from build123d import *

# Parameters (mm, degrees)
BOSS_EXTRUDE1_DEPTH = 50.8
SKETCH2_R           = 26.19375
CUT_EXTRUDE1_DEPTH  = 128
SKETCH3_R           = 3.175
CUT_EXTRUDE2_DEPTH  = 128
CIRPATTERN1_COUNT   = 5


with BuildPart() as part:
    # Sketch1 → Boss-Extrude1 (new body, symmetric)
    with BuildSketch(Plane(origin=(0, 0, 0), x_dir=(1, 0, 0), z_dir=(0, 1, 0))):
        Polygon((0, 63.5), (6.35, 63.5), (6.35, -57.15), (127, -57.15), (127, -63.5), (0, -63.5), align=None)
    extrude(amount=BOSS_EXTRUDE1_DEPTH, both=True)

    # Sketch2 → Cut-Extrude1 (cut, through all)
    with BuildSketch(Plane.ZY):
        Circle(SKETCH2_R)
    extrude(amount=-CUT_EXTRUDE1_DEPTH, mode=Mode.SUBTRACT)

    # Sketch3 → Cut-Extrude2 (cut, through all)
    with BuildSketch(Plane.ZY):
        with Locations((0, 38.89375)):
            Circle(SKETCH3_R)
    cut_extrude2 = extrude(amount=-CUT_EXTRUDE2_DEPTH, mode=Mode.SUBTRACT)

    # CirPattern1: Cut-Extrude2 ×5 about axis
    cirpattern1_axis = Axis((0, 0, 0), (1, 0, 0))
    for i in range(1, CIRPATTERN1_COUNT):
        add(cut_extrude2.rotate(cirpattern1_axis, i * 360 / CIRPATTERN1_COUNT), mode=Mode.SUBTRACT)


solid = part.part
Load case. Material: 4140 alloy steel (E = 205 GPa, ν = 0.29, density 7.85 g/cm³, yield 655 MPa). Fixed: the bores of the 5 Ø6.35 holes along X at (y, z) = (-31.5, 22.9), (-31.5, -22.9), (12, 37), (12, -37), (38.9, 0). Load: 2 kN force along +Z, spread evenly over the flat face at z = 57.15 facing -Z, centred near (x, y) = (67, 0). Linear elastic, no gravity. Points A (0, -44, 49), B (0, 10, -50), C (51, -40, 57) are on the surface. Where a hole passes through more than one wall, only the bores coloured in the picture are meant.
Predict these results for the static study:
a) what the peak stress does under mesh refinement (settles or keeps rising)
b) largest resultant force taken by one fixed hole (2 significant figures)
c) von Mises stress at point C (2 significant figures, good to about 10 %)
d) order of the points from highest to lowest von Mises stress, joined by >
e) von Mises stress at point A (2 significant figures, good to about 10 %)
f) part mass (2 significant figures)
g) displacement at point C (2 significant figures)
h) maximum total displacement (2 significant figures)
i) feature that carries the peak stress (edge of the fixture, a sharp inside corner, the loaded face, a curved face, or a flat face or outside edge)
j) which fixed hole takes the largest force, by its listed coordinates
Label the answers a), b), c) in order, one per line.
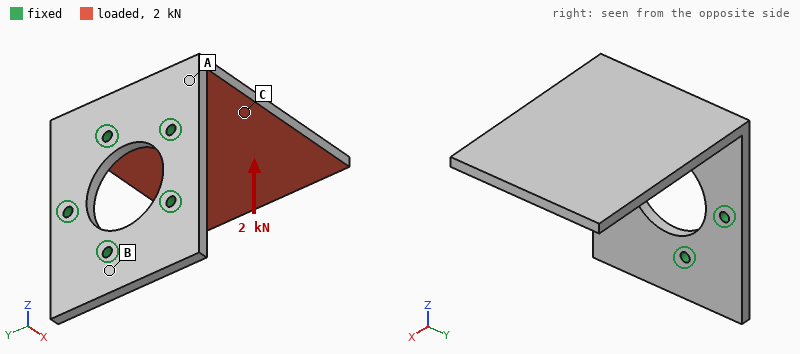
a) keeps rising
b) 2.0 kN
c) 68 MPa
d) A > C > B
e) 150 MPa
f) 1.1 kg
g) 0.60 mm
h) 2.0 mm
i) edge of the fixture
j) (12, 37)
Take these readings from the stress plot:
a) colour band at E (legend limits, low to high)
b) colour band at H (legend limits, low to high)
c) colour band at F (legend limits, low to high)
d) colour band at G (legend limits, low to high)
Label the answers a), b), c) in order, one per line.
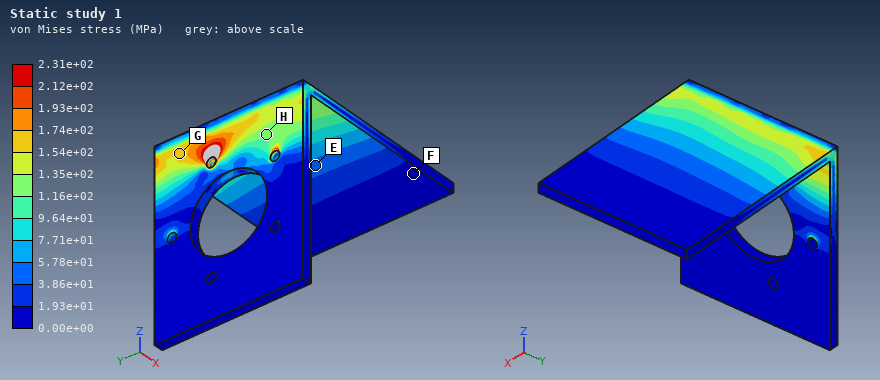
a) 3.86e+01 to 5.78e+01 MPa
b) 1.16e+02 to 1.35e+02 MPa
c) 0.00e+00 to 1.93e+01 MPa
d) 1.54e+02 to 1.74e+02 MPa
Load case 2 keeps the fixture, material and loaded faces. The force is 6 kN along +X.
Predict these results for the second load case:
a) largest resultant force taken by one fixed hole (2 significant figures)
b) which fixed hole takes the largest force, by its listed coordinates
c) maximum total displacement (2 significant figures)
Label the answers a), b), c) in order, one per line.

a) 5.4 kN
b) (12, 37)
c) 0.40 mm
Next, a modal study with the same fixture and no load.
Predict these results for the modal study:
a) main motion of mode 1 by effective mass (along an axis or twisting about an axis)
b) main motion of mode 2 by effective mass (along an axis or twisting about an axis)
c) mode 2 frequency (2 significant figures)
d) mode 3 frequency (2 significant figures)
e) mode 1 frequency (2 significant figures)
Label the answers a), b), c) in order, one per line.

a) along Z
b) along Y
c) 580 Hz
d) 950 Hz
e) 250 Hz
